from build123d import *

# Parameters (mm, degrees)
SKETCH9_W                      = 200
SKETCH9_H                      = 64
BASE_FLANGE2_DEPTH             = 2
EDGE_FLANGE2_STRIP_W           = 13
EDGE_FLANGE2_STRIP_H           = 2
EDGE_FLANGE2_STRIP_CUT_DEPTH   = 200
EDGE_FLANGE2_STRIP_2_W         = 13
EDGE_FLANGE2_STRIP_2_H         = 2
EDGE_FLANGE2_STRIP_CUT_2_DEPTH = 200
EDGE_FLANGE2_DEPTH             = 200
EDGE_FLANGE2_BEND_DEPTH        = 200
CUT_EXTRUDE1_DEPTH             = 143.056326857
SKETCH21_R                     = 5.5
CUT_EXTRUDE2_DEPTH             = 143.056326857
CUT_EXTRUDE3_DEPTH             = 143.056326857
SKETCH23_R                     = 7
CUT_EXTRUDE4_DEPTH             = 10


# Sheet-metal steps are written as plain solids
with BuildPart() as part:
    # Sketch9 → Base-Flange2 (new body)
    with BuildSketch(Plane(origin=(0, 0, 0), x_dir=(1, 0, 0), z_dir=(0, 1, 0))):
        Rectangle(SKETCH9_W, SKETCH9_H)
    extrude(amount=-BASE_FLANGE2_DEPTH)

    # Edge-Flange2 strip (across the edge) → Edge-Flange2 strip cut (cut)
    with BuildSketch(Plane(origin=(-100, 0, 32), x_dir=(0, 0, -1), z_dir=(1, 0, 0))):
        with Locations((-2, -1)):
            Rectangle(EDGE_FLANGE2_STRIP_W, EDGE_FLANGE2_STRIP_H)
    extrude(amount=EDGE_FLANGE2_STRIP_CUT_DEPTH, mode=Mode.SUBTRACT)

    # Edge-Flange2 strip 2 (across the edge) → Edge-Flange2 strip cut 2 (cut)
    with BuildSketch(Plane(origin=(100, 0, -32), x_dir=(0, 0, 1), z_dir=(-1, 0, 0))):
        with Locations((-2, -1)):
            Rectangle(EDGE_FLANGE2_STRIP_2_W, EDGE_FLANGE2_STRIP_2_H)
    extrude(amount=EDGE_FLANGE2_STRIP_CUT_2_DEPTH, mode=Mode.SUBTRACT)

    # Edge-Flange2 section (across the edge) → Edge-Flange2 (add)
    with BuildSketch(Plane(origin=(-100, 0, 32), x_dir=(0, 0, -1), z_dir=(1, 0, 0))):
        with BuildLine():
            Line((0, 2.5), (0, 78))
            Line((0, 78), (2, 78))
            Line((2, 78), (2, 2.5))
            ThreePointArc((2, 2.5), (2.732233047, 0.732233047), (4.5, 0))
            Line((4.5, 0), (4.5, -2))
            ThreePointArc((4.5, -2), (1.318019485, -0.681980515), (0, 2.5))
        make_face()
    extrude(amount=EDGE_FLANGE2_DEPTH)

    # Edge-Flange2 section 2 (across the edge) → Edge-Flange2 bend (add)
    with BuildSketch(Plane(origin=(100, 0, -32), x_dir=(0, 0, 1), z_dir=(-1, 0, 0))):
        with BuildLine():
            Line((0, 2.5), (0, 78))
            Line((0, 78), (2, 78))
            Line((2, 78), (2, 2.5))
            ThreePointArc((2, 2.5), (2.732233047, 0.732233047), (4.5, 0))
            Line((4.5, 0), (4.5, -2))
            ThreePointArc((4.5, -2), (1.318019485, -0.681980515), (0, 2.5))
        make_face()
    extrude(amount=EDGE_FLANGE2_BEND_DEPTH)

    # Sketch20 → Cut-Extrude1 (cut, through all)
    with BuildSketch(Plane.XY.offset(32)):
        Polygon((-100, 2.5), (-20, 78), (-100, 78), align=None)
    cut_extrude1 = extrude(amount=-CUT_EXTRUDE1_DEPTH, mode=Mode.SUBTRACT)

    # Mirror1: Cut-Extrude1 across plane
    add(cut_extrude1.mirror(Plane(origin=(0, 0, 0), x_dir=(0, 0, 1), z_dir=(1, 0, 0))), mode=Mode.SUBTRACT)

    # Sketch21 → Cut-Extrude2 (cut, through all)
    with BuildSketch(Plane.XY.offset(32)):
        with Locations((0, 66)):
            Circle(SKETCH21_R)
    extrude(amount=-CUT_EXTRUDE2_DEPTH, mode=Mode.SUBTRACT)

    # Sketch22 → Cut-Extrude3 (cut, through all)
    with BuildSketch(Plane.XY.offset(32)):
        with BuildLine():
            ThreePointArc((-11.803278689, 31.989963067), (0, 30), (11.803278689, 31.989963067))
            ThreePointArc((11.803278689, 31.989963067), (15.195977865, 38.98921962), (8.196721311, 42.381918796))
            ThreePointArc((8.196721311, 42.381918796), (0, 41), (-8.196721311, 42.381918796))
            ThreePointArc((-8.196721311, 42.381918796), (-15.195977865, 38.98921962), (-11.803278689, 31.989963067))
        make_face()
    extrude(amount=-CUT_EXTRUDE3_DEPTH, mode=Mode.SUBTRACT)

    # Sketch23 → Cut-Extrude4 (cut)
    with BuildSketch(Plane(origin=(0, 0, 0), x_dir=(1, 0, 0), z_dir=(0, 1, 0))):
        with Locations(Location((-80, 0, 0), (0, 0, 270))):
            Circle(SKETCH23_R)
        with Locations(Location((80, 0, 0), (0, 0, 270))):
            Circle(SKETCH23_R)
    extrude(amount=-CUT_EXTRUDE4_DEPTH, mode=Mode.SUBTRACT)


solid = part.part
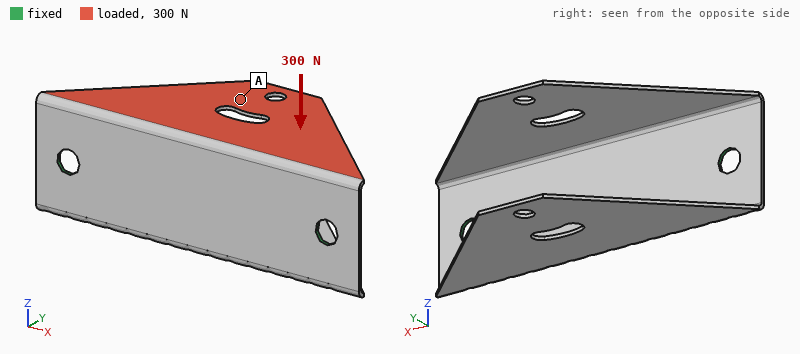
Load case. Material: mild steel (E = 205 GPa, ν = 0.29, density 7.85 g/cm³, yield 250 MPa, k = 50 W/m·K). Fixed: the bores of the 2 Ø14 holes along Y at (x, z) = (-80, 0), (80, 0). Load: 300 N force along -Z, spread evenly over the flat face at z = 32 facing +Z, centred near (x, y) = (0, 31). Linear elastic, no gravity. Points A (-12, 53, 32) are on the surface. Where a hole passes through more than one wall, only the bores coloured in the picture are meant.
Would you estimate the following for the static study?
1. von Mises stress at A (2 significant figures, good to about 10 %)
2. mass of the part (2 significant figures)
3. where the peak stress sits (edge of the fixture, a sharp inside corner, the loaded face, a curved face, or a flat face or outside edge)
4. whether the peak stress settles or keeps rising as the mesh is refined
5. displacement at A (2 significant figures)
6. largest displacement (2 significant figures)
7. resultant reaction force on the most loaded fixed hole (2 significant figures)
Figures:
12 MPa
470 g
edge of the fixture
keeps rising
0.96 mm
1.5 mm
150 N
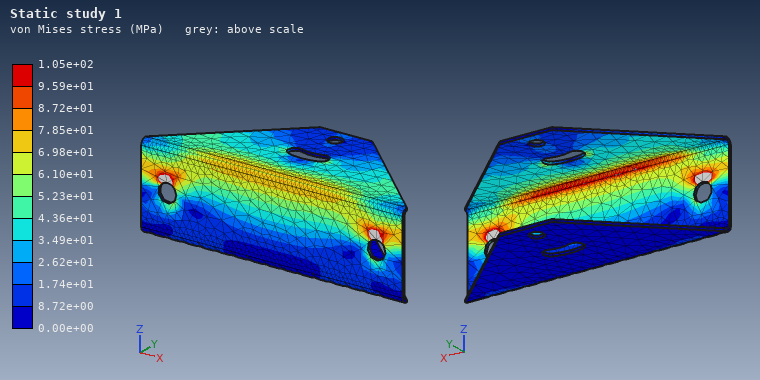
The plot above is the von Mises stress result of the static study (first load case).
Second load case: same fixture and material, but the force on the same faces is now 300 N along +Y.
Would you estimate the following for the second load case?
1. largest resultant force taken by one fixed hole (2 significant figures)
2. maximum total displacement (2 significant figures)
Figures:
170 N
0.42 mm
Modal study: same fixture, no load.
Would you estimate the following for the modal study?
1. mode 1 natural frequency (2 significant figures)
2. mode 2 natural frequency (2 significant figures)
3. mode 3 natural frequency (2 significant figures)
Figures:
250 Hz
260 Hz
640 Hz
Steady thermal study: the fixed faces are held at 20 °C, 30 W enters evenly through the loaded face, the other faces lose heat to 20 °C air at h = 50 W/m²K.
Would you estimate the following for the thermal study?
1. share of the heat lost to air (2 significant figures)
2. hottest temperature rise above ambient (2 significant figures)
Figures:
86 %
47 K
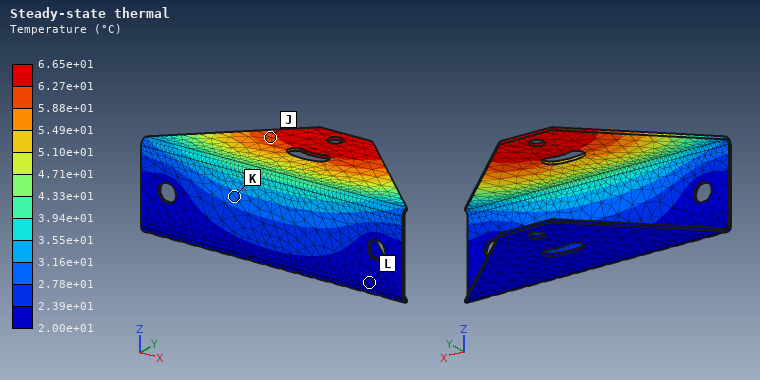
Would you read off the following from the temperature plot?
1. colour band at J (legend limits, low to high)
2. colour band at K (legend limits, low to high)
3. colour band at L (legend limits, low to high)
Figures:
5.88e+01 to 6.27e+01 °C
2.78e+01 to 3.16e+01 °C
2.00e+01 to 2.39e+01 °C
